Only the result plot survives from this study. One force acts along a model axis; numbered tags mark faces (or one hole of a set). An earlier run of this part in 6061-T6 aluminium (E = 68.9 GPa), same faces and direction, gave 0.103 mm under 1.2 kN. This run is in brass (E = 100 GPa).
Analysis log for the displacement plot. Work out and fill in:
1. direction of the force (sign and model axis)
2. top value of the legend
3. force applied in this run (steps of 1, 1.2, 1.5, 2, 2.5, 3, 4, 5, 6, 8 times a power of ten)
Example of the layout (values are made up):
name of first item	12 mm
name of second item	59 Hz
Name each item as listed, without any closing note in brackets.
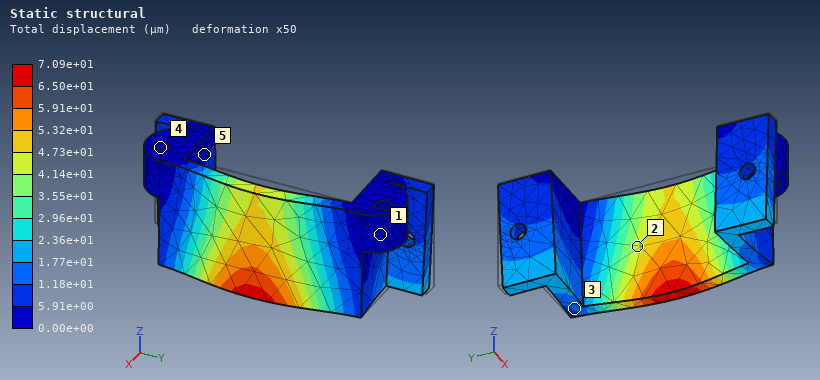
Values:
direction of the force	+X
top value of the legend	7.09e+01 µm
force applied in this run	1.2 kN
